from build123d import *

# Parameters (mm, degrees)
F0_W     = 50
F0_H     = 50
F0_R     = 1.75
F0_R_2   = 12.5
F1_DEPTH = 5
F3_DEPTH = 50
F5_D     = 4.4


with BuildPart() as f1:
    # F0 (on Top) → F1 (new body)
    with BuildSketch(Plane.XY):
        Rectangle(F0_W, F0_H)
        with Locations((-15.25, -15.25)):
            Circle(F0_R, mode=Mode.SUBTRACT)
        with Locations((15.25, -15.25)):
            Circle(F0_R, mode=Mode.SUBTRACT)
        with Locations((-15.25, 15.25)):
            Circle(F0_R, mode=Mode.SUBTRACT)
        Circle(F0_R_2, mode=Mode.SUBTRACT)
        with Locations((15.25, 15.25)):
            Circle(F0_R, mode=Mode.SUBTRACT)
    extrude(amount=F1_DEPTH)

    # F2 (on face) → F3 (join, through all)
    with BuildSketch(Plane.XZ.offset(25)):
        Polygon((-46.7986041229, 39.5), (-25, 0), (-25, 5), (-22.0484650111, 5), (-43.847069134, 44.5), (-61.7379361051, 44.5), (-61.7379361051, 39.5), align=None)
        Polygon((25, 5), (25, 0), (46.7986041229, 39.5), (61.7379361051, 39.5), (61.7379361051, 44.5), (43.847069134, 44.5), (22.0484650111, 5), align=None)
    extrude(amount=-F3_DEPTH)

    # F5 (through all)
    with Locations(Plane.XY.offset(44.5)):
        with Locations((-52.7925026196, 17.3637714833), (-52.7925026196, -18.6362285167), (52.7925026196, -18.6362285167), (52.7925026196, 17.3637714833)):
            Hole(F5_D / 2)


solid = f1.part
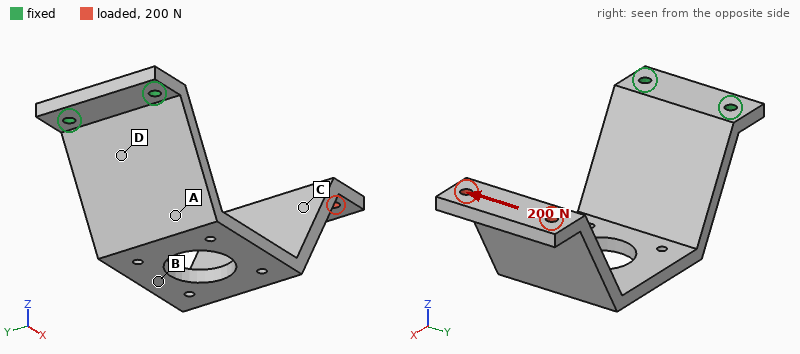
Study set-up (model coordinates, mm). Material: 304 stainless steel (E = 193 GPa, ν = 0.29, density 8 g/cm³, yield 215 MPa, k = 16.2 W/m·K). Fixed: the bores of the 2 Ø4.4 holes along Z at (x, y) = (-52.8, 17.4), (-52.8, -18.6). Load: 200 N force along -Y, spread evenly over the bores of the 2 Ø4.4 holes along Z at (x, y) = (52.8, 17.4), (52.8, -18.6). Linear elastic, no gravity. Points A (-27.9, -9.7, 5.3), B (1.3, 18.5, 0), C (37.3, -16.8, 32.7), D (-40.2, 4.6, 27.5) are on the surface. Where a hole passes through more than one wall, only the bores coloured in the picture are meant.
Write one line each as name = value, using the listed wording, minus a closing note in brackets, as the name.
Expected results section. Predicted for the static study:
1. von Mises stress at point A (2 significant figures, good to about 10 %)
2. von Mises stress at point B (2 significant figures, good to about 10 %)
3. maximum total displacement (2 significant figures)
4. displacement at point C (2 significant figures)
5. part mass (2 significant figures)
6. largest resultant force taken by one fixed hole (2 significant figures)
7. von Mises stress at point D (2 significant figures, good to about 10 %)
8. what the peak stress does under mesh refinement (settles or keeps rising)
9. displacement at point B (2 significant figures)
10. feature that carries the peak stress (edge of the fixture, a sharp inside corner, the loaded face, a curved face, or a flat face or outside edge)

von Mises stress at point A = 62 MPa
von Mises stress at point B = 45 MPa
maximum total displacement = 0.56 mm
displacement at point C = 0.40 mm
part mass = 320 g
largest resultant force taken by one fixed hole = 570 N
von Mises stress at point D = 58 MPa
what the peak stress does under mesh refinement = keeps rising
displacement at point B = 0.13 mm
feature that carries the peak stress = edge of the fixture
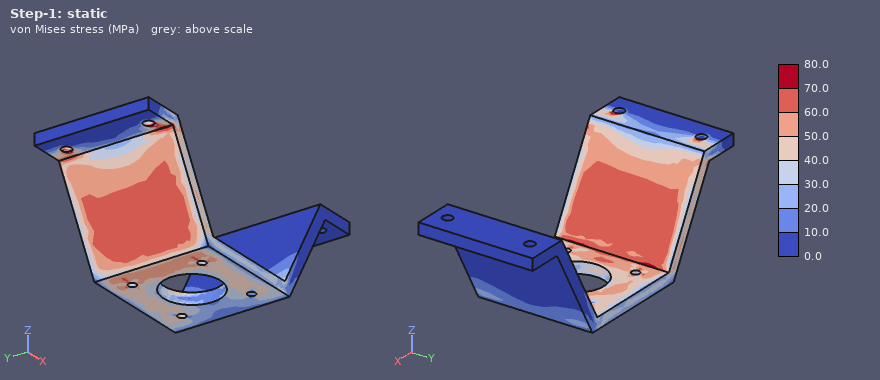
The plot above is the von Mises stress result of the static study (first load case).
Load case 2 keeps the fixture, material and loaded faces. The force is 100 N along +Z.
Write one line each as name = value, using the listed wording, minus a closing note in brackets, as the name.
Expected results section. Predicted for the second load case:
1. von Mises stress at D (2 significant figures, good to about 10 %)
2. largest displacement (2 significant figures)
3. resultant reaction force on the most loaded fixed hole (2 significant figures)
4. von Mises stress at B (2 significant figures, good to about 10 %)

von Mises stress at D = 40 MPa
largest displacement = 0.77 mm
resultant reaction force on the most loaded fixed hole = 56 N
von Mises stress at B = 48 MPa
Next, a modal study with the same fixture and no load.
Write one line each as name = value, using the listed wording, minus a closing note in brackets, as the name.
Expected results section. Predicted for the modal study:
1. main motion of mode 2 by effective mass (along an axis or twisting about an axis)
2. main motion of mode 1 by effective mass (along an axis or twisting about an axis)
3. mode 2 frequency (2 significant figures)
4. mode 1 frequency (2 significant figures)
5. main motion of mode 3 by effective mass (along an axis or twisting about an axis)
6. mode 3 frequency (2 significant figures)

main motion of mode 2 by effective mass = along Y
main motion of mode 1 by effective mass = along Z
mode 2 frequency = 350 Hz
mode 1 frequency = 200 Hz
main motion of mode 3 by effective mass = along X
mode 3 frequency = 560 Hz
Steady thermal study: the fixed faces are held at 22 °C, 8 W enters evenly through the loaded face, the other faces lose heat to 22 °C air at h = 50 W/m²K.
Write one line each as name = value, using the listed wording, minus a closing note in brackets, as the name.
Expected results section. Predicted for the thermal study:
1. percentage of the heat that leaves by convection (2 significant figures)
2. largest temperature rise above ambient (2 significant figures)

percentage of the heat that leaves by convection = 100 %
largest temperature rise above ambient = 50 K
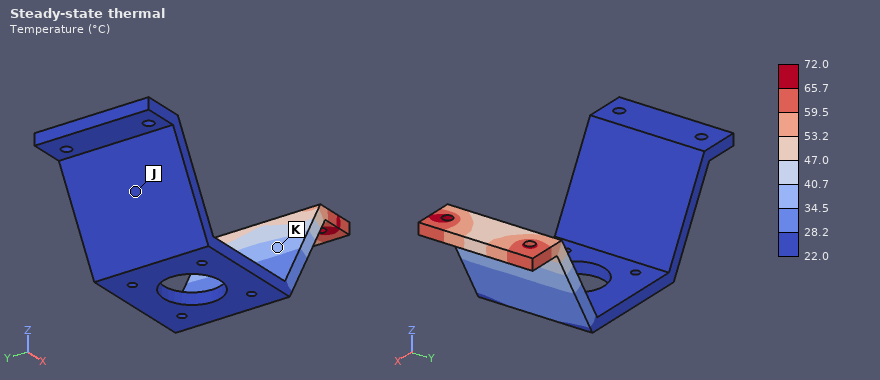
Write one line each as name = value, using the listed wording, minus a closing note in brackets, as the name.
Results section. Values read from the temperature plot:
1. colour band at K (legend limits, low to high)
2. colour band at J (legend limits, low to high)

colour band at K = 34.5 to 40.7 °C
colour band at J = 22.0 to 28.2 °C
